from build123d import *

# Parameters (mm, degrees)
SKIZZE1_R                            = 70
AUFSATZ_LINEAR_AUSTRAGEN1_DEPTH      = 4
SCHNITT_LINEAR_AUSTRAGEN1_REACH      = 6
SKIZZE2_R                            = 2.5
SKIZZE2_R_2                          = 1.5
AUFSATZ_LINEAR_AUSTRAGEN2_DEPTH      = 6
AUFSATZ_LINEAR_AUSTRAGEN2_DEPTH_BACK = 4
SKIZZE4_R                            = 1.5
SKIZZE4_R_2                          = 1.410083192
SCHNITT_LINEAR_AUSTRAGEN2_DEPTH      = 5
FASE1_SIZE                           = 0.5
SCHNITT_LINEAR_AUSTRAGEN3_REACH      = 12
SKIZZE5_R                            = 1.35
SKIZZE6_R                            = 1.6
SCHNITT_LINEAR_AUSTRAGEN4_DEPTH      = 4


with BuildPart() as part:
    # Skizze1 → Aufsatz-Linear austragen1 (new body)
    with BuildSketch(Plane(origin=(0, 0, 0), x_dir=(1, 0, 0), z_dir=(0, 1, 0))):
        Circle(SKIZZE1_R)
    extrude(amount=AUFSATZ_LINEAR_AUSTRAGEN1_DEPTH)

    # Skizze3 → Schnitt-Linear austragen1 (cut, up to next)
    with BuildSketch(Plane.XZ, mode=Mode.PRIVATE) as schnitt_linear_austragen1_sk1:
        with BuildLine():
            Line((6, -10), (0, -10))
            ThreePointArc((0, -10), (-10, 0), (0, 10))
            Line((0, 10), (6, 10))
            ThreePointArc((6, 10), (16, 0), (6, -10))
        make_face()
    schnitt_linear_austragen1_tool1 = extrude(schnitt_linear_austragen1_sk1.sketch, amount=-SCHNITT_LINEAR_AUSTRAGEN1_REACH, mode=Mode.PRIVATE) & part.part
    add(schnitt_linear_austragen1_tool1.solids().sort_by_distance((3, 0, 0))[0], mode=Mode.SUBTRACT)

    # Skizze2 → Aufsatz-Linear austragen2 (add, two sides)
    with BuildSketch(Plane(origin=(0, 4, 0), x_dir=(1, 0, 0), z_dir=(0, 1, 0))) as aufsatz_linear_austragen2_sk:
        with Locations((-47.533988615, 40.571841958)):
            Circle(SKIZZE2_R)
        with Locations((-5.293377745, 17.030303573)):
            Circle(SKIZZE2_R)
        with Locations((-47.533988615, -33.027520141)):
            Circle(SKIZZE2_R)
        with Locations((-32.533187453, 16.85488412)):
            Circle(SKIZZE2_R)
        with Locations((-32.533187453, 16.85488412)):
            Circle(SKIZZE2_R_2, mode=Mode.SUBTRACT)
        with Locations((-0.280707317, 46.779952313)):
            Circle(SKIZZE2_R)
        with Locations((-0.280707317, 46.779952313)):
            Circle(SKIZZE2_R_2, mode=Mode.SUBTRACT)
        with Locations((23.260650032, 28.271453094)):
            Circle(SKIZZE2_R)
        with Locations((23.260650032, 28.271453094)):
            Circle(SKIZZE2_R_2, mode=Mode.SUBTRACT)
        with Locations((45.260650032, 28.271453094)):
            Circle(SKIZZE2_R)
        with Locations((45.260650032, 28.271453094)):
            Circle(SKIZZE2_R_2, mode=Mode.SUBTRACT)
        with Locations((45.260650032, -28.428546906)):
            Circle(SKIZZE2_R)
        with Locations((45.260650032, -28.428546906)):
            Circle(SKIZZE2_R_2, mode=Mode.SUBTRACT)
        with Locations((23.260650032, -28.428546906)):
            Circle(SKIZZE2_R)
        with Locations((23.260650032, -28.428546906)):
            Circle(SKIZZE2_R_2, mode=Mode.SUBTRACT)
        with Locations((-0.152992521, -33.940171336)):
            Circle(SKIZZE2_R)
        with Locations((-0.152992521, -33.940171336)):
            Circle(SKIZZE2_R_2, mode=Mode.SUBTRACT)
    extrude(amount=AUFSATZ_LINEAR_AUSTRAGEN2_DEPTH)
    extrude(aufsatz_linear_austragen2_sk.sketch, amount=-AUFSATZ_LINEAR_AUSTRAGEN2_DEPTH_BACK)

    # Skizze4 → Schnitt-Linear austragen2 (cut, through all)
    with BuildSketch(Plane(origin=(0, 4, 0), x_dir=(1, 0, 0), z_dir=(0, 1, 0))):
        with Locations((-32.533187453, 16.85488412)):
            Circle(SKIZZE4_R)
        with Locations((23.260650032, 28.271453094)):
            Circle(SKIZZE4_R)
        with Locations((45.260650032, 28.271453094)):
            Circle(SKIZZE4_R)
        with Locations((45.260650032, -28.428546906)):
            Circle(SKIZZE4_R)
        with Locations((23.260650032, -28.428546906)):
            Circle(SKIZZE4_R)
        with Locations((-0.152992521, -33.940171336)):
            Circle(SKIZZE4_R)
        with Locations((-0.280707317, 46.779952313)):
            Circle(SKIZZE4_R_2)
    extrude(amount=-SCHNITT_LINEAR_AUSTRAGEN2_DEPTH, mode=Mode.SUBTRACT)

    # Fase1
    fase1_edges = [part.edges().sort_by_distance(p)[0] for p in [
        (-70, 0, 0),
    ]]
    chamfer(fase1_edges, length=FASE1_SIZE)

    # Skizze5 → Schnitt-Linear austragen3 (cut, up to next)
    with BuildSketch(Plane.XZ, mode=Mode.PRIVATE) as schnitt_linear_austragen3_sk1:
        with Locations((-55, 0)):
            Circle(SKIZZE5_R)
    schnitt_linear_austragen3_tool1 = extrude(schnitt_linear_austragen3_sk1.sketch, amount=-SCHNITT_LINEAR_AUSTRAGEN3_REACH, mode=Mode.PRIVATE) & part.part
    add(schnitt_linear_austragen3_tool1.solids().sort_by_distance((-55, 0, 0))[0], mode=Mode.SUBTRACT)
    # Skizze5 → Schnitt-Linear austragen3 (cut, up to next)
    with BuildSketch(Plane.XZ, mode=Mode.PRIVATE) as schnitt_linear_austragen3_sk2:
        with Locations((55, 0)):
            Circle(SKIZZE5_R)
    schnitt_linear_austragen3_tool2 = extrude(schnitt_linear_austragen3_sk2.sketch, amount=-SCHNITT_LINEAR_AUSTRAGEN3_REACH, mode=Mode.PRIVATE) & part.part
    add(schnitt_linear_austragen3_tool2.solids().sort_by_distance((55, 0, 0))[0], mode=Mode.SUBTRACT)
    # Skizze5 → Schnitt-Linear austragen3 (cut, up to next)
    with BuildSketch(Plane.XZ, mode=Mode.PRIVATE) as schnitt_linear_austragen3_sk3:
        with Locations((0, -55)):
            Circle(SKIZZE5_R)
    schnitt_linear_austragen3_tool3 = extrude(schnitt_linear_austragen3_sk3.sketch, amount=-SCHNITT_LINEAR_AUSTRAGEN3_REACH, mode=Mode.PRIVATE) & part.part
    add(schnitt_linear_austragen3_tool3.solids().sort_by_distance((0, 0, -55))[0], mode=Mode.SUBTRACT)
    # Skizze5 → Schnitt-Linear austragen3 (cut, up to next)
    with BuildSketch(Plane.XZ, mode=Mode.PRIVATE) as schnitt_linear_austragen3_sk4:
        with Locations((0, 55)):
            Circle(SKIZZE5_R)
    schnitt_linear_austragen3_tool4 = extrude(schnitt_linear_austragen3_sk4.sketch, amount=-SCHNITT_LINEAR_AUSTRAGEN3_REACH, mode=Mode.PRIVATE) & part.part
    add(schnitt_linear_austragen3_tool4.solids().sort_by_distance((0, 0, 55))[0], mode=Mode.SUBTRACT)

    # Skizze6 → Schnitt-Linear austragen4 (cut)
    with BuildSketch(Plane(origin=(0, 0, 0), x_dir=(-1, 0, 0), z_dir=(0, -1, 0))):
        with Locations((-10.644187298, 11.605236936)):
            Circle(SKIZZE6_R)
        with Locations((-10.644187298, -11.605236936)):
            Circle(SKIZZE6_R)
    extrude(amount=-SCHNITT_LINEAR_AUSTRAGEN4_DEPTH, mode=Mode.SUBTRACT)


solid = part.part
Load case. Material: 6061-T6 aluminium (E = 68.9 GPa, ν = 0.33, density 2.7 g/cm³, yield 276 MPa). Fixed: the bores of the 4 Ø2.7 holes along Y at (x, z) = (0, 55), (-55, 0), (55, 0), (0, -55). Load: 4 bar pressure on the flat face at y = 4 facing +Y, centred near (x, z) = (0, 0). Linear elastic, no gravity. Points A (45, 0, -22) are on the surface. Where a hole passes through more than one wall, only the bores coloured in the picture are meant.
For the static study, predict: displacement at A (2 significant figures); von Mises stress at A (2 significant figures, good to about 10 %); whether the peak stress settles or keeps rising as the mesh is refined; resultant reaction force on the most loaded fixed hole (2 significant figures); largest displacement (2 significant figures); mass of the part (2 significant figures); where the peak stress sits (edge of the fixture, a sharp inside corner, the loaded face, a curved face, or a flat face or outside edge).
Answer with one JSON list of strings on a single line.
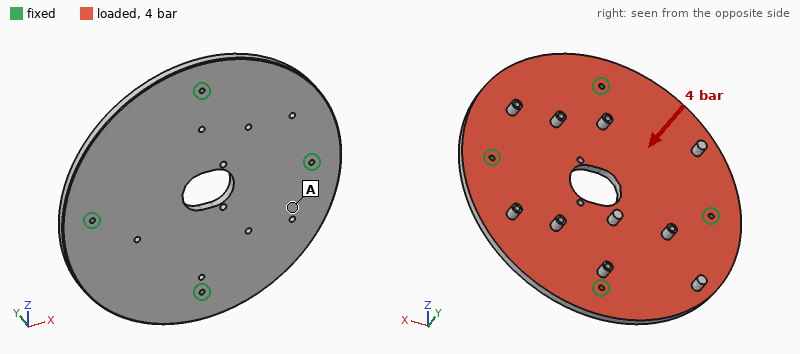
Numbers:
["0.12 mm", "37 MPa", "keeps rising", "1.5 kN", "0.27 mm", "160 g", "edge of the fixture"]
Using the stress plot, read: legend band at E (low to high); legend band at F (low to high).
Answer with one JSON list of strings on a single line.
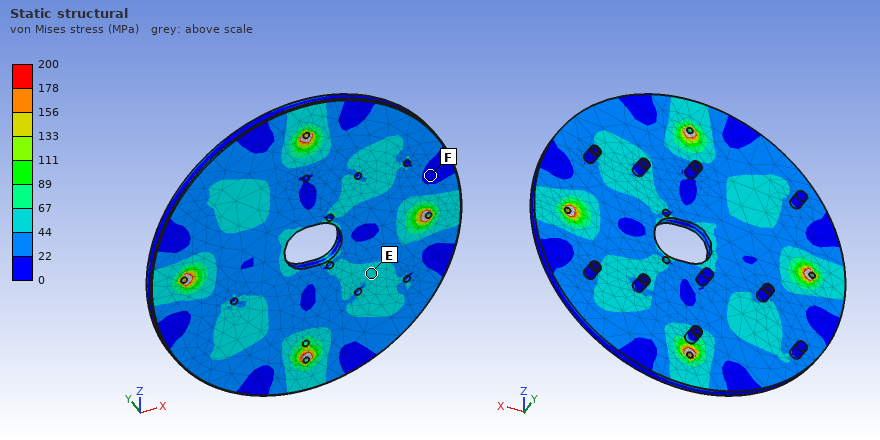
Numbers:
["44 to 67 MPa", "0 to 22 MPa"]
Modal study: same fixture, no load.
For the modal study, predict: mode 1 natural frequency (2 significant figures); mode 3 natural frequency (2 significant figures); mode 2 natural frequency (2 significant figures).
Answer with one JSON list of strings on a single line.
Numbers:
["1900 Hz", "2200 Hz", "2200 Hz"]
